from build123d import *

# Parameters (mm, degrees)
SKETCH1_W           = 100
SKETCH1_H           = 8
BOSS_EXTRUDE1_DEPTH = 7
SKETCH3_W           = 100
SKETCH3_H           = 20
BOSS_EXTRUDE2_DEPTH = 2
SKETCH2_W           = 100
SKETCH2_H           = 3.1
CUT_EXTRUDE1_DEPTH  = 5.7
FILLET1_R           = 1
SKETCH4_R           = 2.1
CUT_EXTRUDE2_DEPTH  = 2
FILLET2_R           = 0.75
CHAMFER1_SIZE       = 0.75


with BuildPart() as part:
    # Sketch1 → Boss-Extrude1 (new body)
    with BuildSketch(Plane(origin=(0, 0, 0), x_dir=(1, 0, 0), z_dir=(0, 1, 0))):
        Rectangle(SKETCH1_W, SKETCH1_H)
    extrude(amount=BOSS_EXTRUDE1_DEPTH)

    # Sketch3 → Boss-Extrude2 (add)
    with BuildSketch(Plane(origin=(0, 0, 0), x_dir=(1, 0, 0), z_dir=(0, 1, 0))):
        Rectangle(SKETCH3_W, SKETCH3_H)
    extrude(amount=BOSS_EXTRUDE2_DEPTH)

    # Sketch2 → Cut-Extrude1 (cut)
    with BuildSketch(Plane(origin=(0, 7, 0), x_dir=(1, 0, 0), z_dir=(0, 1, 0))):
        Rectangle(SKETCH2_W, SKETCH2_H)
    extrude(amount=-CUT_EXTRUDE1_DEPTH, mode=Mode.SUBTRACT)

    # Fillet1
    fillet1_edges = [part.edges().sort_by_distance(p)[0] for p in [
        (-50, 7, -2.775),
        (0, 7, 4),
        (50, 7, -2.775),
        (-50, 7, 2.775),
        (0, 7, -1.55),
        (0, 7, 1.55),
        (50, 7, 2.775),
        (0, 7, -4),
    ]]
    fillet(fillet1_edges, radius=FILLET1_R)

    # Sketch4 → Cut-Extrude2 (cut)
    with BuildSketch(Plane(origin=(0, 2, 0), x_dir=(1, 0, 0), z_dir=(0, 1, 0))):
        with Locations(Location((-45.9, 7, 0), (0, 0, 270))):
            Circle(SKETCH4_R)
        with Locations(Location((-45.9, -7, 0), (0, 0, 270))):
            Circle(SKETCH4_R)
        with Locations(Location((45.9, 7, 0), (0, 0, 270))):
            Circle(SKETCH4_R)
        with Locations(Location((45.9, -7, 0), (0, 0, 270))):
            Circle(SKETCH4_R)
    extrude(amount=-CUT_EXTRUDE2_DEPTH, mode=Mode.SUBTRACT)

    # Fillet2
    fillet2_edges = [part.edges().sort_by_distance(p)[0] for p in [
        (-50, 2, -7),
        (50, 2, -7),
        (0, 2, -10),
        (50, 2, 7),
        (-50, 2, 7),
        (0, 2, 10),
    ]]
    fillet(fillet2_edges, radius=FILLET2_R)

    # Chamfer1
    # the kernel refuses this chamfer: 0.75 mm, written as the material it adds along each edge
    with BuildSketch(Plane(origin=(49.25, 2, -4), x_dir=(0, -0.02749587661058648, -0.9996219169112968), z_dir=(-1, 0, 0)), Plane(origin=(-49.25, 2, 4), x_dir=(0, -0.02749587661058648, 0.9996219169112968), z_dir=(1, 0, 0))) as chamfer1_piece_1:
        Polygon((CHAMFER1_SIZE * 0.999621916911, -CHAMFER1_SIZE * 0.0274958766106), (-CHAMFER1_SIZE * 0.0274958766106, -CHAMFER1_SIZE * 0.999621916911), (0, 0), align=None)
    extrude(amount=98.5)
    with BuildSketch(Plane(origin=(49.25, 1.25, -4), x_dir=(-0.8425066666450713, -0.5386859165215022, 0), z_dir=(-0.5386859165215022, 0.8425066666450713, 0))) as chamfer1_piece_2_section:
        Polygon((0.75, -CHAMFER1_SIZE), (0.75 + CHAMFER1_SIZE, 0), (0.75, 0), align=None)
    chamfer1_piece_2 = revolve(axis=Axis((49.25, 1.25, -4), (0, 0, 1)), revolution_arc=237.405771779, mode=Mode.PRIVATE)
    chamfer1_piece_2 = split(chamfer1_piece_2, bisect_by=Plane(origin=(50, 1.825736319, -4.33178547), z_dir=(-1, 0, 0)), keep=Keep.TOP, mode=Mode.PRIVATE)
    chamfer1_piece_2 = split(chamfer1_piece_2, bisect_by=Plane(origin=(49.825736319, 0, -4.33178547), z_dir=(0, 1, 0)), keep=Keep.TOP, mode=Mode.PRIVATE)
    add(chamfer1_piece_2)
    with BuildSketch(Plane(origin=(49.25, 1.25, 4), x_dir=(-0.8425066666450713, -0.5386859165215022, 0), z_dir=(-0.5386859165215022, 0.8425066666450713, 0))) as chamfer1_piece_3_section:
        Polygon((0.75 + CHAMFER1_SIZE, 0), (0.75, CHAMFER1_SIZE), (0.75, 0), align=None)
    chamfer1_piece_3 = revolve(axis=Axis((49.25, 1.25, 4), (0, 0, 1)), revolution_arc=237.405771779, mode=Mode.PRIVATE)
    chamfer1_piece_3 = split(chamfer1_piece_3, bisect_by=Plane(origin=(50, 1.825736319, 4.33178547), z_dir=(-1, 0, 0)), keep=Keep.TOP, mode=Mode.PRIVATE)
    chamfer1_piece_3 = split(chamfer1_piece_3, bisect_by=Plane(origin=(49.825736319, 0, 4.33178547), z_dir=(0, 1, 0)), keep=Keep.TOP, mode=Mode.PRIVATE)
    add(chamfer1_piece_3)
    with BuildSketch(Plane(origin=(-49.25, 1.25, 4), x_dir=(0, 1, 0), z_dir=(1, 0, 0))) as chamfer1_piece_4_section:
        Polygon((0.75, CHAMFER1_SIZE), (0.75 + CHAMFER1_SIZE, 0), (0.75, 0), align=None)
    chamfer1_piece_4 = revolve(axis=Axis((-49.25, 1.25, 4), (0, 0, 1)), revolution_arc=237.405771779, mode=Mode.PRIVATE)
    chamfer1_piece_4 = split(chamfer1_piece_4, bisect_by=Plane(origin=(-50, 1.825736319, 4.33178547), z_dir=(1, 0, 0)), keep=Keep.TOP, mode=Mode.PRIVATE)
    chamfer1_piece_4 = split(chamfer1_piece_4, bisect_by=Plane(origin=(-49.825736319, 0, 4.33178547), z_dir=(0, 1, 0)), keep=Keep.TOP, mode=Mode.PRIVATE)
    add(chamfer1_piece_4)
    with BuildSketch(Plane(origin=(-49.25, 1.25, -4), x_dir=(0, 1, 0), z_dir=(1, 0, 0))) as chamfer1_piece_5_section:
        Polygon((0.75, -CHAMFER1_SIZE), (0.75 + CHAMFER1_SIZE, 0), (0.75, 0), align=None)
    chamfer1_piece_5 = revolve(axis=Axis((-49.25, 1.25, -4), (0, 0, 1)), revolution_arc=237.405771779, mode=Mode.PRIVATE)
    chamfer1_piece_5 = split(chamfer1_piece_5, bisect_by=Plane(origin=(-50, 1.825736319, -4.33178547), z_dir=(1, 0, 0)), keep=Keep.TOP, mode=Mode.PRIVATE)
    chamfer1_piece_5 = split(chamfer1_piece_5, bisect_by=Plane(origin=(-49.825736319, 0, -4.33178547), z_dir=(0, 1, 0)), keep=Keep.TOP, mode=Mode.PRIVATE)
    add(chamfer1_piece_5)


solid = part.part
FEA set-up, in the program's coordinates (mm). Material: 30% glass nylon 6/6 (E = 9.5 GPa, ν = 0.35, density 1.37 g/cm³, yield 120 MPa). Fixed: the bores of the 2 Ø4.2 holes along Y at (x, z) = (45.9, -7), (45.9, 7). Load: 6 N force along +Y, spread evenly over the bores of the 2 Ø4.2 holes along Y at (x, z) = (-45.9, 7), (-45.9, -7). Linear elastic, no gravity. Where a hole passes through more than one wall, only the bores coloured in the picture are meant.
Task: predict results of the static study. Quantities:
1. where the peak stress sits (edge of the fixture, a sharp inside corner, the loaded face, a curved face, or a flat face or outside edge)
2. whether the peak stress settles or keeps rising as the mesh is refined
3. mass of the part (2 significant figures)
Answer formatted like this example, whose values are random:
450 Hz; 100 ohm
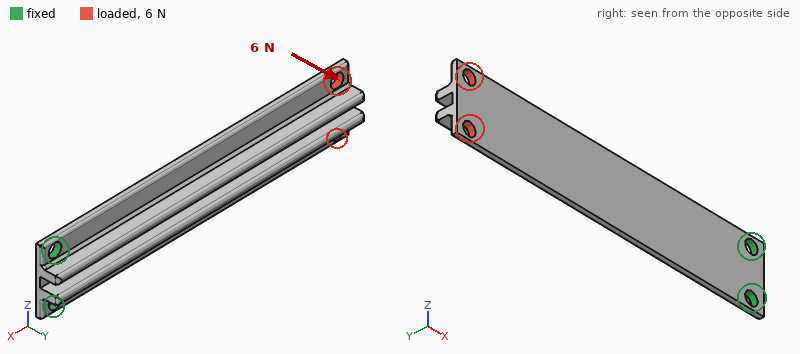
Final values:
edge of the fixture; keeps rising; 8.3 g
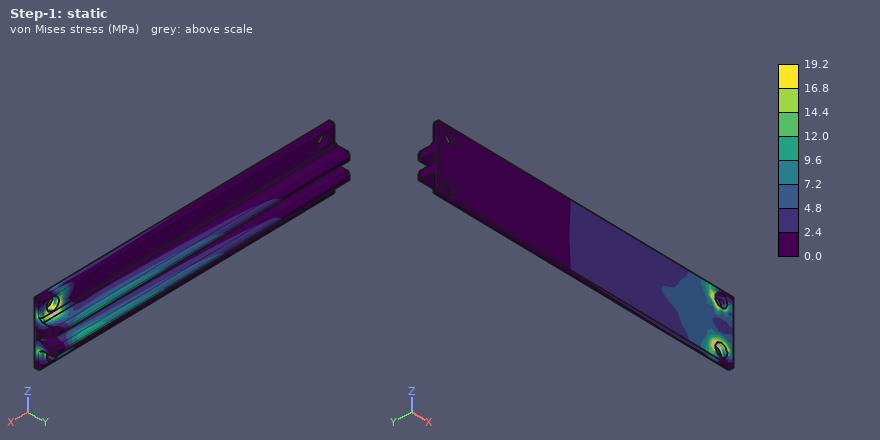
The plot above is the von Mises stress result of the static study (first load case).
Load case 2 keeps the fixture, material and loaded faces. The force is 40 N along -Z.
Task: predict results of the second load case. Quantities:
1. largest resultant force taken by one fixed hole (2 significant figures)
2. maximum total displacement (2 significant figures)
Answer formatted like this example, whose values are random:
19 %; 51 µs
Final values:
250 N; 0.80 mm
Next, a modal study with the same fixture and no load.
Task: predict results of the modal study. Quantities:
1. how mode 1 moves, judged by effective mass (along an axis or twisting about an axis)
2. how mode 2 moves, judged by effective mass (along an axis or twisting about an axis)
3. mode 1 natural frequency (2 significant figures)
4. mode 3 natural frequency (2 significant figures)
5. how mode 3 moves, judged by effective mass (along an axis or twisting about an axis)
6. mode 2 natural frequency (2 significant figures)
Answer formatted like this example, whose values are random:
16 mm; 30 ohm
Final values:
along Y; along Z; 250 Hz; 1100 Hz; twisting about X; 760 Hz
